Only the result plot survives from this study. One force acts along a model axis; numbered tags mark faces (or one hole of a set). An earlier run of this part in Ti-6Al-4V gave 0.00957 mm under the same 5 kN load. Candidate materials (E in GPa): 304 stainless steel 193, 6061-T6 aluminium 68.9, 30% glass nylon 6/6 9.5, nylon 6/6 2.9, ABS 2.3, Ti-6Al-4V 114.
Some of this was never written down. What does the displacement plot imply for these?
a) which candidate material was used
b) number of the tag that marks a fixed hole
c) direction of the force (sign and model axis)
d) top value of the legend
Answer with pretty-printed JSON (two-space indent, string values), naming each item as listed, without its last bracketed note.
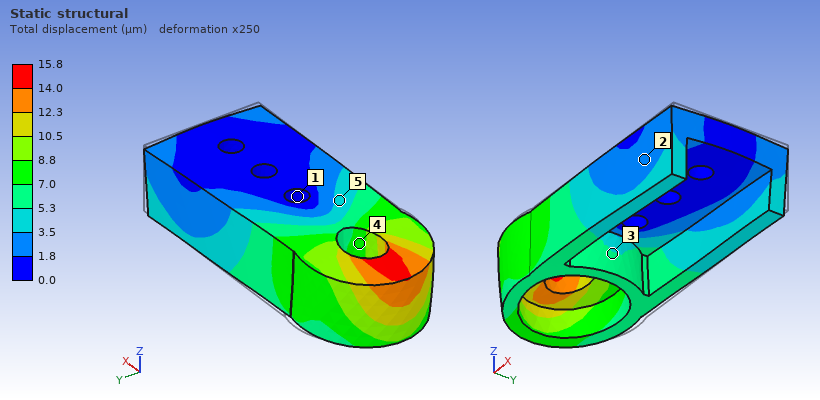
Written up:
{
  "which candidate material was used": "6061-T6 aluminium",
  "number of the tag that marks a fixed hole": "1",
  "direction of the force": "-X",
  "top value of the legend": "15.8 µm"
}
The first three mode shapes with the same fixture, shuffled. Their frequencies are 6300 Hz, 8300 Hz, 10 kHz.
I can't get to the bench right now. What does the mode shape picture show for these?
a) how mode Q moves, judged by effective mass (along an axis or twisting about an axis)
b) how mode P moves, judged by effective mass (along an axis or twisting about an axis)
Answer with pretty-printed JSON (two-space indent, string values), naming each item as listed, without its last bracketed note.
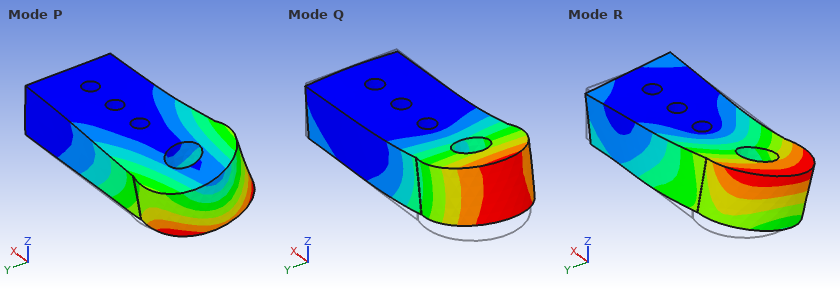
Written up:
{
  "how mode Q moves, judged by effective mass": "along Z",
  "how mode P moves, judged by effective mass": "along Y"
}
